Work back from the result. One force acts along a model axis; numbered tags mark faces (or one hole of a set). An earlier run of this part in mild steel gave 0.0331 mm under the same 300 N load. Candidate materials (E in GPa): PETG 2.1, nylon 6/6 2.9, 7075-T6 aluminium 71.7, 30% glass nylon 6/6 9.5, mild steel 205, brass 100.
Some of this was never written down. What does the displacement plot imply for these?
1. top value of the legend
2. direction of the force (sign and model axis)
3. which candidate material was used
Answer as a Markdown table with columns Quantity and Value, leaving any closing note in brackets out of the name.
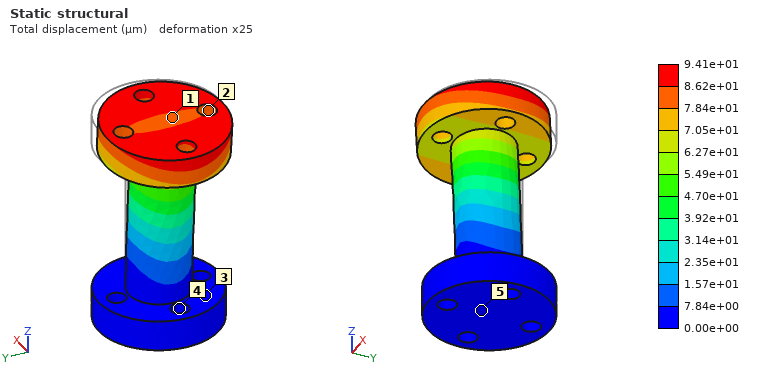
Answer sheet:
| Quantity | Value |
|---|---|
| top value of the legend | 9.41e+01 µm |
| direction of the force | -X |
| which candidate material was used | 7075-T6 aluminium |
